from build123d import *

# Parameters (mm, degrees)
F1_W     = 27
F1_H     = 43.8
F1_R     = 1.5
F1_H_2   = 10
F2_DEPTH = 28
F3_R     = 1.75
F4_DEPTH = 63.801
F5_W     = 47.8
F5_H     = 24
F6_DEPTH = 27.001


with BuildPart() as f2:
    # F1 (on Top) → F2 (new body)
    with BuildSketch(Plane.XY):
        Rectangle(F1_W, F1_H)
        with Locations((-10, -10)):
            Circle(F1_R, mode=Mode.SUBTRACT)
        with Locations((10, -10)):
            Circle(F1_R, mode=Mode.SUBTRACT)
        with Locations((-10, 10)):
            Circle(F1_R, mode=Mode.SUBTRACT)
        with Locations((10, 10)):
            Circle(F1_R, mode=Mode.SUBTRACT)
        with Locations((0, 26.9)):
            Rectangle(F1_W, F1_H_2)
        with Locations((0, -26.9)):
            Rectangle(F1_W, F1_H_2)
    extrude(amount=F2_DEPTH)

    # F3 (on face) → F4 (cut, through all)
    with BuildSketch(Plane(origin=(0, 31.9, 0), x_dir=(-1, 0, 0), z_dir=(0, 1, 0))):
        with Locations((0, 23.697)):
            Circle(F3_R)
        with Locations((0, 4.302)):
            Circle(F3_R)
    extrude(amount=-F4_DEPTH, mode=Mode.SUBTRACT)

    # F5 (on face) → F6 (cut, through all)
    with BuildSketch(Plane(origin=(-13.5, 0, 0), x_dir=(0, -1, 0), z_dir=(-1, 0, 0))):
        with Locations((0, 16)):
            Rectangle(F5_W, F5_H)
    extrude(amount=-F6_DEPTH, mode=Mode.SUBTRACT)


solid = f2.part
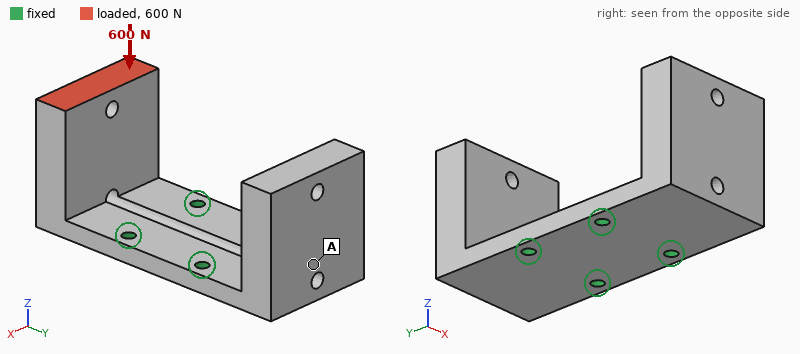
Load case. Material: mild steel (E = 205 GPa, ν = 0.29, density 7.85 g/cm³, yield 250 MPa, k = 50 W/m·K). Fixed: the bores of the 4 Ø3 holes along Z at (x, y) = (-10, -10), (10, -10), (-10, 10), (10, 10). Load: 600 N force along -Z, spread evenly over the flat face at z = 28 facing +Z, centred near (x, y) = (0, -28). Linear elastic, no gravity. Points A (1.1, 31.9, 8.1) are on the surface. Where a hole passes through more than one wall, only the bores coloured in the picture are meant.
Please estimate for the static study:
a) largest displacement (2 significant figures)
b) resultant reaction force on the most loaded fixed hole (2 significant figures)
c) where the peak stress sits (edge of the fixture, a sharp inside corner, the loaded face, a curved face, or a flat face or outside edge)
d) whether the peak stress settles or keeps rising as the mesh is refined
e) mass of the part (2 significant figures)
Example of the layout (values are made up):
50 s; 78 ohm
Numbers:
0.11 mm; 360 N; edge of the fixture; keeps rising; 130 g
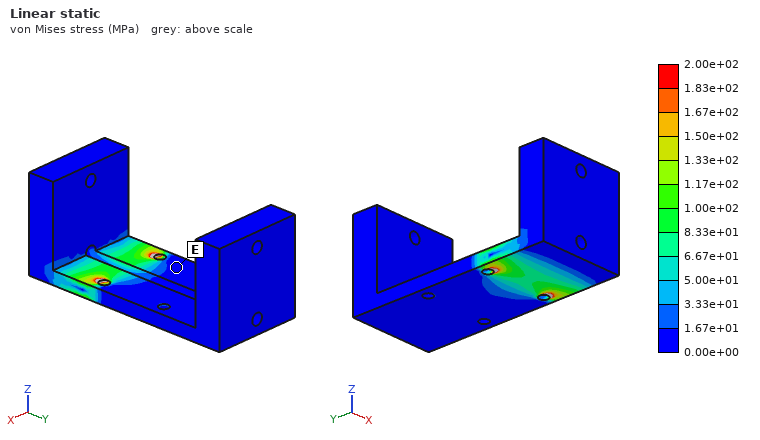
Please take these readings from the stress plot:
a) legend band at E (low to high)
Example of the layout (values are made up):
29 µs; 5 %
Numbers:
0.00e+00 to 1.67e+01 MPa
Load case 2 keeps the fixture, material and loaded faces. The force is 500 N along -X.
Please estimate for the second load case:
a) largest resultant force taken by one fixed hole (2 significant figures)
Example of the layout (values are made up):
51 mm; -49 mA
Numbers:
780 N
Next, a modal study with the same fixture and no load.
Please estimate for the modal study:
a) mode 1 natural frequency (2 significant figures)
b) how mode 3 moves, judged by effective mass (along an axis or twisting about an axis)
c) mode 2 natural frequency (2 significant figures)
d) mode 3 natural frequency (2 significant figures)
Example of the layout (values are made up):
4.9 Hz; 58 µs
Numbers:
1700 Hz; along X; 1700 Hz; 3600 Hz
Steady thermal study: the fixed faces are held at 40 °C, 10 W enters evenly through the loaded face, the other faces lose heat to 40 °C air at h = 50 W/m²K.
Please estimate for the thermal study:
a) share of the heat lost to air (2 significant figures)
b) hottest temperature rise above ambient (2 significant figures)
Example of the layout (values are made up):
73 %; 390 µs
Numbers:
37 %; 42 K
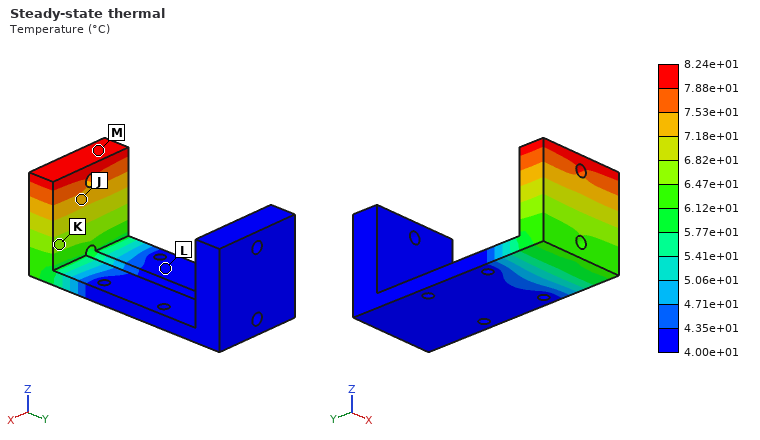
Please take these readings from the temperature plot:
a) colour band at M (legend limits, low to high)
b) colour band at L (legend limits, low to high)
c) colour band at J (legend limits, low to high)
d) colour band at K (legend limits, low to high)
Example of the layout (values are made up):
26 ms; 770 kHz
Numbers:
7.88e+01 to 8.24e+01 °C; 4.00e+01 to 4.35e+01 °C; 7.18e+01 to 7.53e+01 °C; 6.47e+01 to 6.82e+01 °C
